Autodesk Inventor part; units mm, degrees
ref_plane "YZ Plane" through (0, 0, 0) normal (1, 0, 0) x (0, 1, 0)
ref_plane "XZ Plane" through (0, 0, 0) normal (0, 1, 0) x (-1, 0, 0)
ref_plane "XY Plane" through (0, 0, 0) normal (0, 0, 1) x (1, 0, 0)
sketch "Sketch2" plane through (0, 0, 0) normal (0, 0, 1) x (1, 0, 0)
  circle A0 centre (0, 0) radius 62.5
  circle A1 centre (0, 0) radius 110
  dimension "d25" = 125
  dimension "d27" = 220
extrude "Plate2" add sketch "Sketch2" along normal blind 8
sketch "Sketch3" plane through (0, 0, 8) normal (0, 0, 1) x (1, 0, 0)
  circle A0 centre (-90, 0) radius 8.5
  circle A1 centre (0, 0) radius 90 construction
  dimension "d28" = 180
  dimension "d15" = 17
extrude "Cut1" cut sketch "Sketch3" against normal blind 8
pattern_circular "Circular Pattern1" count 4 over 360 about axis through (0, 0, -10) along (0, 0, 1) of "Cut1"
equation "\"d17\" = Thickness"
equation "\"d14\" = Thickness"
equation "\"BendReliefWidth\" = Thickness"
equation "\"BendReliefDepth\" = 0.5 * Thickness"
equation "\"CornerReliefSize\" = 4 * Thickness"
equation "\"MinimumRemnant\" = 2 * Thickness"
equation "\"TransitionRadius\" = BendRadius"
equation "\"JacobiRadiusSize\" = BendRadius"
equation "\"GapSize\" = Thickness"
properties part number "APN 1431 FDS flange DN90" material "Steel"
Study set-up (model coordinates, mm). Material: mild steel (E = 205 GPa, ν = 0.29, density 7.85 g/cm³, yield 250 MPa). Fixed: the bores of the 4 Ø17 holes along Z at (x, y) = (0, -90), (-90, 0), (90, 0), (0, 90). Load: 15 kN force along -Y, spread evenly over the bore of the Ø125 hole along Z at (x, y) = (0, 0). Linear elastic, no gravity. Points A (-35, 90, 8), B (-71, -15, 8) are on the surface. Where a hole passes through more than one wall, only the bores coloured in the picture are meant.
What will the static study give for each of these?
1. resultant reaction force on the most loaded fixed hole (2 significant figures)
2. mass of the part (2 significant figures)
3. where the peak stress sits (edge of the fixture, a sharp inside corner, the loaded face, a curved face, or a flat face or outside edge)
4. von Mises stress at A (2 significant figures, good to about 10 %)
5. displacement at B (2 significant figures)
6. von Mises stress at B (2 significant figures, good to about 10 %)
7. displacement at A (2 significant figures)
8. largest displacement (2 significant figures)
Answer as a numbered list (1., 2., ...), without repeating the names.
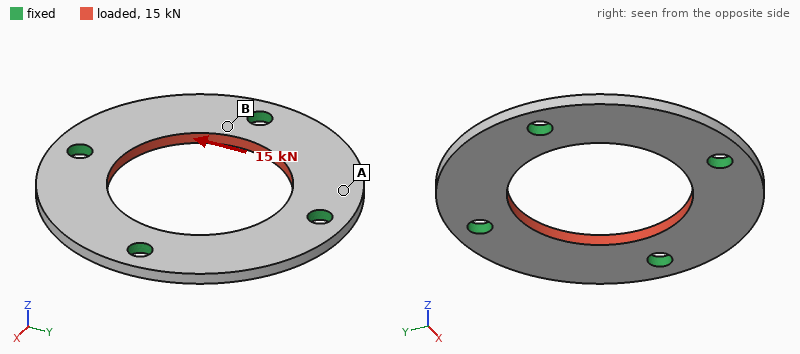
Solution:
1. 4.3 kN
2. 1.6 kg
3. edge of the fixture
4. 4.0 MPa
5. 1.7 µm
6. 8.4 MPa
7. 1.7 µm
8. 3.2 µm
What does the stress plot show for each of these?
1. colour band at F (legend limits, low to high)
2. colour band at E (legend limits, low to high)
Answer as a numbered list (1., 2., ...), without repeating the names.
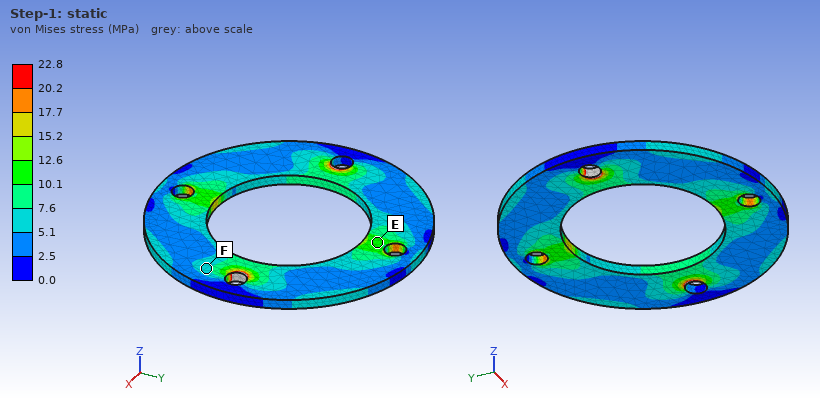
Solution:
1. 5.1 to 7.6 MPa
2. 10.1 to 12.6 MPa
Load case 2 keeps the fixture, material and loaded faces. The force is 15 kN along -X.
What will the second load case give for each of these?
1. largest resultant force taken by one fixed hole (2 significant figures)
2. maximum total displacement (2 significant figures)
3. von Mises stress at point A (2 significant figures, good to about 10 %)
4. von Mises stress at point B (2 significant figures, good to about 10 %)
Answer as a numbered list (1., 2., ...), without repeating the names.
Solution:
1. 4.3 kN
2. 3.2 µm
3. 5.1 MPa
4. 9.7 MPa
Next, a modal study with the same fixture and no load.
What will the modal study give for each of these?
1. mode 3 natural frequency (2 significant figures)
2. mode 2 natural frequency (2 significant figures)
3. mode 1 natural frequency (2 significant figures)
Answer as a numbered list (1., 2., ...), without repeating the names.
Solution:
1. 2200 Hz
2. 2200 Hz
3. 2200 Hz
